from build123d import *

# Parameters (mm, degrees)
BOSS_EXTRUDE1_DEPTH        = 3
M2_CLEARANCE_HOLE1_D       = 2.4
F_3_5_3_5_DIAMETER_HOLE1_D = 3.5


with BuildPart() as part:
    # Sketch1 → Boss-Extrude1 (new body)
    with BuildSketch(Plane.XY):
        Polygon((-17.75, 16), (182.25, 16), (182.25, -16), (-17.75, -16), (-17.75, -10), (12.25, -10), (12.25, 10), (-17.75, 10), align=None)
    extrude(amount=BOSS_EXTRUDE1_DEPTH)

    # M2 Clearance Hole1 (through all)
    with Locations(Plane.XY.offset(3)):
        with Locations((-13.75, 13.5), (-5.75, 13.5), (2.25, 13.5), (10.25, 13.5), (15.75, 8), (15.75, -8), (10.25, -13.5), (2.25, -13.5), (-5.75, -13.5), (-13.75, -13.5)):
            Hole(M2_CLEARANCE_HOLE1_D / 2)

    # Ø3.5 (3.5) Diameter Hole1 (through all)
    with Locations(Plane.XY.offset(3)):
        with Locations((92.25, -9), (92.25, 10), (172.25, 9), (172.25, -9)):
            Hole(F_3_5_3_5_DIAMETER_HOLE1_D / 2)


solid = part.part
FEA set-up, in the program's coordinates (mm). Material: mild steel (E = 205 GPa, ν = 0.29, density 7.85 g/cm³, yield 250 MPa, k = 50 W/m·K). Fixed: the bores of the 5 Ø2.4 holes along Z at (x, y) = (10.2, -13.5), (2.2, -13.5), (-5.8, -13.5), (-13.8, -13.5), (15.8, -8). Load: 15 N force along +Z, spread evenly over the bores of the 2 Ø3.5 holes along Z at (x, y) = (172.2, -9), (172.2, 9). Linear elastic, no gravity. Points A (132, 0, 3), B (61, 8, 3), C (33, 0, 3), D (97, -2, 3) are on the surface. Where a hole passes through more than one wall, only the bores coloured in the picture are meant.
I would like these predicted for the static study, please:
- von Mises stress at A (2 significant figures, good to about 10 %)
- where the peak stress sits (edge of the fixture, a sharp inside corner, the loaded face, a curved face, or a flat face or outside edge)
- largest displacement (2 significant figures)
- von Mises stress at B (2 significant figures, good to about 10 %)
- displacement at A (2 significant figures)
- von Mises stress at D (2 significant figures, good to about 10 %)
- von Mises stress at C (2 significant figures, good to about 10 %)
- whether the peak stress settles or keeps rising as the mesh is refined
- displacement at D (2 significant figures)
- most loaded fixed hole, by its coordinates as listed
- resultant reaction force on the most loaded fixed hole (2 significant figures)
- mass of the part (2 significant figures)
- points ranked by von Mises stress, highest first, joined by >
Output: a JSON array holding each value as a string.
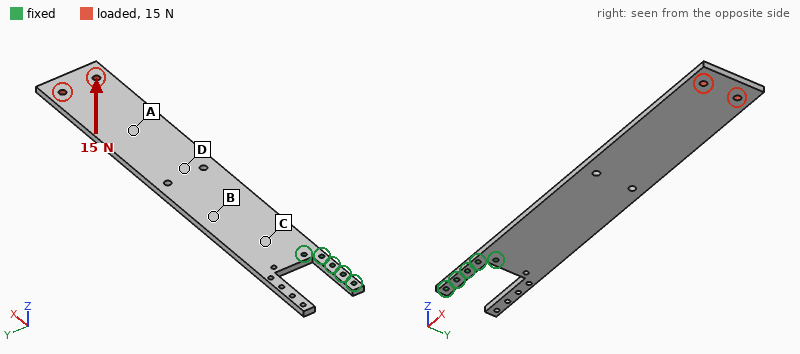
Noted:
["13 MPa", "edge of the fixture", "1.6 mm", "35 MPa", "0.95 mm", "25 MPa", "42 MPa", "keeps rising", "0.53 mm", "(15.8, -8)", "100 N", "130 g", "C > B > D > A"]
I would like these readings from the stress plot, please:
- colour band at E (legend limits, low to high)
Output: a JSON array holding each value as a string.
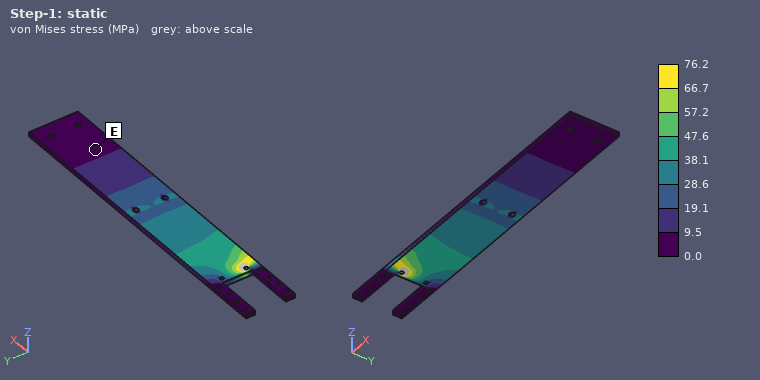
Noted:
["0.0 to 9.5 MPa"]
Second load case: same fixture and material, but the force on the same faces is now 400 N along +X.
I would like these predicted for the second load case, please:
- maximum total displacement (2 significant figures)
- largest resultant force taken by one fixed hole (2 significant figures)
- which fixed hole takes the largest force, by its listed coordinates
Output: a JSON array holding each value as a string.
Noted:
["65 µm", "690 N", "(15.8, -8)"]
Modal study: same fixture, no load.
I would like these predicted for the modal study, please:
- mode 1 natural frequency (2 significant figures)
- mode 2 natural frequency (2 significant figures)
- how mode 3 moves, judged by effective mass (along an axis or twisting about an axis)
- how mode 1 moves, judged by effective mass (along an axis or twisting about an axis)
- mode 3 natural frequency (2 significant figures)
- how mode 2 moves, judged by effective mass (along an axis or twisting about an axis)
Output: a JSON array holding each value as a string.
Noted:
["83 Hz", "420 Hz", "along Z", "along Z", "520 Hz", "along Y"]
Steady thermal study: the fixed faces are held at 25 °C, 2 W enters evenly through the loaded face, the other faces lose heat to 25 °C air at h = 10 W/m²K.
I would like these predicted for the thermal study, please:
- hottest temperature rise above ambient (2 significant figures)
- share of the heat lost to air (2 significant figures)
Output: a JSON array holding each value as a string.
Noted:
["31 K", "78 %"]
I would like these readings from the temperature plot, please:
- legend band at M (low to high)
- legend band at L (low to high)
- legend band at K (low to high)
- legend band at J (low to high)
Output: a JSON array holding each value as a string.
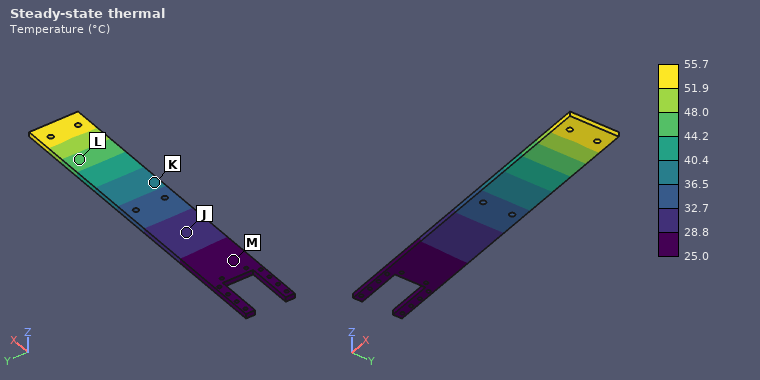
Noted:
["25.0 to 28.8 °C", "44.2 to 48.0 °C", "36.5 to 40.4 °C", "28.8 to 32.7 °C"]
